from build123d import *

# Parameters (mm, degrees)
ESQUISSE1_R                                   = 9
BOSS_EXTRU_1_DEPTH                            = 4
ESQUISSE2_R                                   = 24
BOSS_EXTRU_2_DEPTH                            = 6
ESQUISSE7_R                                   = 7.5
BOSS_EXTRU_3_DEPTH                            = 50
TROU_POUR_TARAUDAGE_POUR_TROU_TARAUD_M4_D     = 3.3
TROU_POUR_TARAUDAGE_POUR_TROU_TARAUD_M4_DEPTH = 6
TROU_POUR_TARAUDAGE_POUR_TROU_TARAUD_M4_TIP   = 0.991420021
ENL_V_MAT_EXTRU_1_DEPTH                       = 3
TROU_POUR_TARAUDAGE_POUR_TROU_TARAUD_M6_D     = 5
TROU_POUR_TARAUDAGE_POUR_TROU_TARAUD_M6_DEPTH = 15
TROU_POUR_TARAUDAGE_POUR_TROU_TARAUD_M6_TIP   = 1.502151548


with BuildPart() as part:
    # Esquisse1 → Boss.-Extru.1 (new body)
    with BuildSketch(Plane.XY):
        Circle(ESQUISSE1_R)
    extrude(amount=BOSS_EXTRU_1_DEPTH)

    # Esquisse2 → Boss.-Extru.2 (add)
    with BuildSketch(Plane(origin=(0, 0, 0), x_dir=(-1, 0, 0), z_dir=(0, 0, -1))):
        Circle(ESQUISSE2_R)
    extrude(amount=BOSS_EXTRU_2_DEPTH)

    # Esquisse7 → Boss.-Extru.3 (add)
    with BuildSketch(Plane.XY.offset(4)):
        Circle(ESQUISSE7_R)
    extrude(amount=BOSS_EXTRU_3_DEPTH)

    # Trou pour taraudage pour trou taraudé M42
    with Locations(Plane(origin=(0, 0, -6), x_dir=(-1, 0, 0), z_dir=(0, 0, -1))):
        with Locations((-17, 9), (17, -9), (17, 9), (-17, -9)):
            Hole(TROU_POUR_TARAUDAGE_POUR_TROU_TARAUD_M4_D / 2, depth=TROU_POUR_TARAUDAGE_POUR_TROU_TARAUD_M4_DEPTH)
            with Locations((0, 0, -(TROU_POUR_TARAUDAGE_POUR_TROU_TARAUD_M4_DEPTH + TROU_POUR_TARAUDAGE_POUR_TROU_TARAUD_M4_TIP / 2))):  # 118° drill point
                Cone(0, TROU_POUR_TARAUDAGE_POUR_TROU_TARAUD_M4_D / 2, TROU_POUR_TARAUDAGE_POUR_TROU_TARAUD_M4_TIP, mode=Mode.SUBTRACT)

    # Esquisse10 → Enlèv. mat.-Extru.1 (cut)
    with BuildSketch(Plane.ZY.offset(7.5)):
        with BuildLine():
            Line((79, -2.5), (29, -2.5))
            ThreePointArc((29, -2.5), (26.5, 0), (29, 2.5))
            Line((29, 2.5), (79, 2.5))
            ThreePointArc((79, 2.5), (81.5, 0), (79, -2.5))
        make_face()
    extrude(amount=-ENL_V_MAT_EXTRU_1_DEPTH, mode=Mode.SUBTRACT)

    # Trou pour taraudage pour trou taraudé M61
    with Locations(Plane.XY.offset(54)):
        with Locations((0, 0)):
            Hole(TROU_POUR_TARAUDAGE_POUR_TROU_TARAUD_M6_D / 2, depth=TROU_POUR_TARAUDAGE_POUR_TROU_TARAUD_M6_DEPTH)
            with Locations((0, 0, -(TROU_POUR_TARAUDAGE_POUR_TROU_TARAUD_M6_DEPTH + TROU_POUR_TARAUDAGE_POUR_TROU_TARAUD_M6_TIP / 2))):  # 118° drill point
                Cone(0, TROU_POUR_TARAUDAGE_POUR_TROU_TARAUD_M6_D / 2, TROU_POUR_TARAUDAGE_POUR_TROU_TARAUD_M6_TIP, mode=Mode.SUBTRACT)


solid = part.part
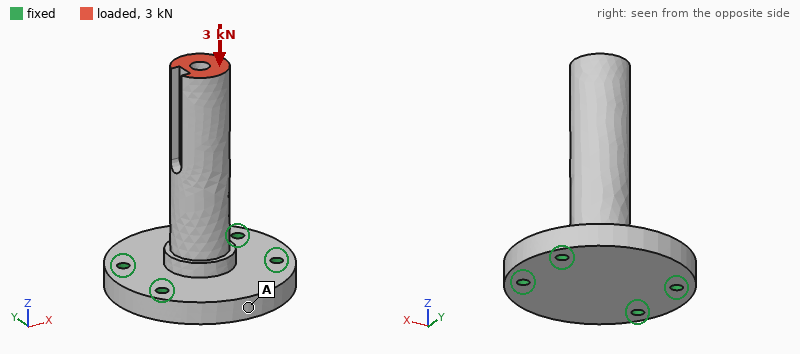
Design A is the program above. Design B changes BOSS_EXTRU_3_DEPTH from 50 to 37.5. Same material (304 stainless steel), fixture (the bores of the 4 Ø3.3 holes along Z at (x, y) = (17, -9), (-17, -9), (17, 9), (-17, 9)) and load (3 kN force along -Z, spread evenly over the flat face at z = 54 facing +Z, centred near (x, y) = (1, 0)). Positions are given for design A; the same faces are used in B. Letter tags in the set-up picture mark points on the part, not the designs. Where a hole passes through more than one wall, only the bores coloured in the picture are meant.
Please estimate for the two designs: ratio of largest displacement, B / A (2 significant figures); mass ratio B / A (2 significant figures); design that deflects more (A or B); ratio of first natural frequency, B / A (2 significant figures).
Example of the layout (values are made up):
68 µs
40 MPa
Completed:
0.85
0.91
A
1.5
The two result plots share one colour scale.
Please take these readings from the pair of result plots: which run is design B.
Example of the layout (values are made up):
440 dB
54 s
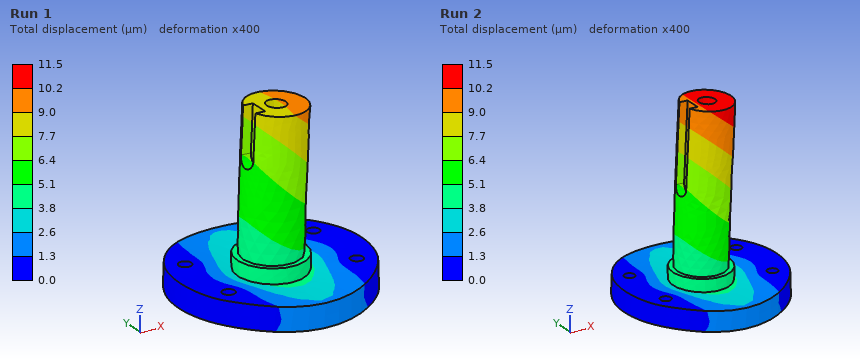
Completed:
Run 1
